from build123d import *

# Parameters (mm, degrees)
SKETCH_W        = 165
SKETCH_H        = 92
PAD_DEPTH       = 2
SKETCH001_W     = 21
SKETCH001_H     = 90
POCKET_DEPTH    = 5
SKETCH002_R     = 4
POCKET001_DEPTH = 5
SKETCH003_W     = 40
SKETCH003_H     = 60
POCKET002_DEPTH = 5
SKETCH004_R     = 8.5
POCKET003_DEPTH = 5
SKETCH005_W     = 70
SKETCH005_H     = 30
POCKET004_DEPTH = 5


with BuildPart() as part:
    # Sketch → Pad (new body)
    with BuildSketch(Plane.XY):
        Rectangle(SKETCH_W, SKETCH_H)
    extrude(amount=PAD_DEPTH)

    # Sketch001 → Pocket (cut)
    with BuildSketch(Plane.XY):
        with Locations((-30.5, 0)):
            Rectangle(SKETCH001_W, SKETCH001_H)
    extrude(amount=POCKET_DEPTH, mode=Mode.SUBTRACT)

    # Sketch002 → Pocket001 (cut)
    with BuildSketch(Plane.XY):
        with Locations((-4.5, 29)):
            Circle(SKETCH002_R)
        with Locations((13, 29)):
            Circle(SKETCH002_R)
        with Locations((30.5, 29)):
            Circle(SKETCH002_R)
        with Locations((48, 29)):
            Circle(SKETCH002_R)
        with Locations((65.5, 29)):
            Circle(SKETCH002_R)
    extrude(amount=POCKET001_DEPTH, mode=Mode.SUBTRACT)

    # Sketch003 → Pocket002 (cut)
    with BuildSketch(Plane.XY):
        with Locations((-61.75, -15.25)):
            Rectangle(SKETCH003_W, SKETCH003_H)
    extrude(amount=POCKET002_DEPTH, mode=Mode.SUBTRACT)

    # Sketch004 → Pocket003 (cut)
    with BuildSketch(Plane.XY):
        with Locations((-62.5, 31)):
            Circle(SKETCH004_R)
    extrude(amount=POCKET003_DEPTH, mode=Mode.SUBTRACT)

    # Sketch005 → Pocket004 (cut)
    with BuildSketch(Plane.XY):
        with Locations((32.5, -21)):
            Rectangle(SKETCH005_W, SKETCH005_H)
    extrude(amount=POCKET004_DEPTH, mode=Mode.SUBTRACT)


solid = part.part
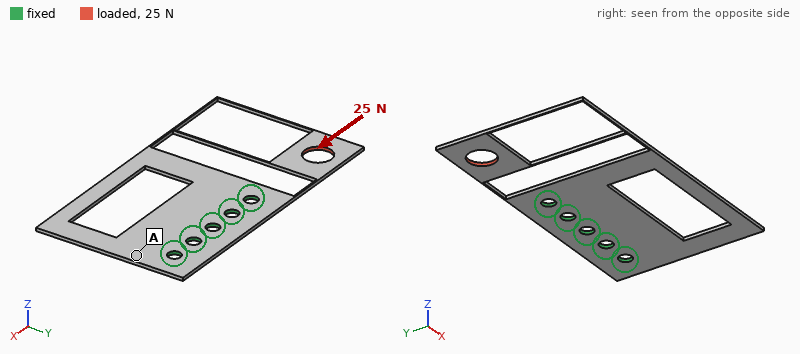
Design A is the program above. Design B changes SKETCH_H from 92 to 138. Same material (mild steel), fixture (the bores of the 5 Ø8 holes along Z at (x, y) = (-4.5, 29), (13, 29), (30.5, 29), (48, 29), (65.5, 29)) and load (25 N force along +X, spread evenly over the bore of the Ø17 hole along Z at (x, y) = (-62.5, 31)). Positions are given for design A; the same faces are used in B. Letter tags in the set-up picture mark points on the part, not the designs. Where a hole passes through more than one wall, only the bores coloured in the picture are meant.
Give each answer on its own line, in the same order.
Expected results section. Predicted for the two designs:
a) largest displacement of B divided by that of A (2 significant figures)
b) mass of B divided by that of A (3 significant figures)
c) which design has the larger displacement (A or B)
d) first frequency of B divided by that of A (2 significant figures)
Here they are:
0.0017
1.91
A
1.2
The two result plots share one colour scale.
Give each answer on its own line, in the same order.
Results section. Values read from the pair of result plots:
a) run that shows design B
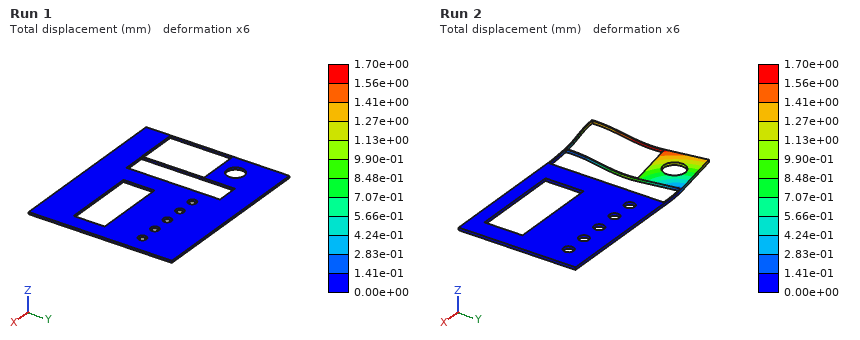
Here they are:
Run 1
